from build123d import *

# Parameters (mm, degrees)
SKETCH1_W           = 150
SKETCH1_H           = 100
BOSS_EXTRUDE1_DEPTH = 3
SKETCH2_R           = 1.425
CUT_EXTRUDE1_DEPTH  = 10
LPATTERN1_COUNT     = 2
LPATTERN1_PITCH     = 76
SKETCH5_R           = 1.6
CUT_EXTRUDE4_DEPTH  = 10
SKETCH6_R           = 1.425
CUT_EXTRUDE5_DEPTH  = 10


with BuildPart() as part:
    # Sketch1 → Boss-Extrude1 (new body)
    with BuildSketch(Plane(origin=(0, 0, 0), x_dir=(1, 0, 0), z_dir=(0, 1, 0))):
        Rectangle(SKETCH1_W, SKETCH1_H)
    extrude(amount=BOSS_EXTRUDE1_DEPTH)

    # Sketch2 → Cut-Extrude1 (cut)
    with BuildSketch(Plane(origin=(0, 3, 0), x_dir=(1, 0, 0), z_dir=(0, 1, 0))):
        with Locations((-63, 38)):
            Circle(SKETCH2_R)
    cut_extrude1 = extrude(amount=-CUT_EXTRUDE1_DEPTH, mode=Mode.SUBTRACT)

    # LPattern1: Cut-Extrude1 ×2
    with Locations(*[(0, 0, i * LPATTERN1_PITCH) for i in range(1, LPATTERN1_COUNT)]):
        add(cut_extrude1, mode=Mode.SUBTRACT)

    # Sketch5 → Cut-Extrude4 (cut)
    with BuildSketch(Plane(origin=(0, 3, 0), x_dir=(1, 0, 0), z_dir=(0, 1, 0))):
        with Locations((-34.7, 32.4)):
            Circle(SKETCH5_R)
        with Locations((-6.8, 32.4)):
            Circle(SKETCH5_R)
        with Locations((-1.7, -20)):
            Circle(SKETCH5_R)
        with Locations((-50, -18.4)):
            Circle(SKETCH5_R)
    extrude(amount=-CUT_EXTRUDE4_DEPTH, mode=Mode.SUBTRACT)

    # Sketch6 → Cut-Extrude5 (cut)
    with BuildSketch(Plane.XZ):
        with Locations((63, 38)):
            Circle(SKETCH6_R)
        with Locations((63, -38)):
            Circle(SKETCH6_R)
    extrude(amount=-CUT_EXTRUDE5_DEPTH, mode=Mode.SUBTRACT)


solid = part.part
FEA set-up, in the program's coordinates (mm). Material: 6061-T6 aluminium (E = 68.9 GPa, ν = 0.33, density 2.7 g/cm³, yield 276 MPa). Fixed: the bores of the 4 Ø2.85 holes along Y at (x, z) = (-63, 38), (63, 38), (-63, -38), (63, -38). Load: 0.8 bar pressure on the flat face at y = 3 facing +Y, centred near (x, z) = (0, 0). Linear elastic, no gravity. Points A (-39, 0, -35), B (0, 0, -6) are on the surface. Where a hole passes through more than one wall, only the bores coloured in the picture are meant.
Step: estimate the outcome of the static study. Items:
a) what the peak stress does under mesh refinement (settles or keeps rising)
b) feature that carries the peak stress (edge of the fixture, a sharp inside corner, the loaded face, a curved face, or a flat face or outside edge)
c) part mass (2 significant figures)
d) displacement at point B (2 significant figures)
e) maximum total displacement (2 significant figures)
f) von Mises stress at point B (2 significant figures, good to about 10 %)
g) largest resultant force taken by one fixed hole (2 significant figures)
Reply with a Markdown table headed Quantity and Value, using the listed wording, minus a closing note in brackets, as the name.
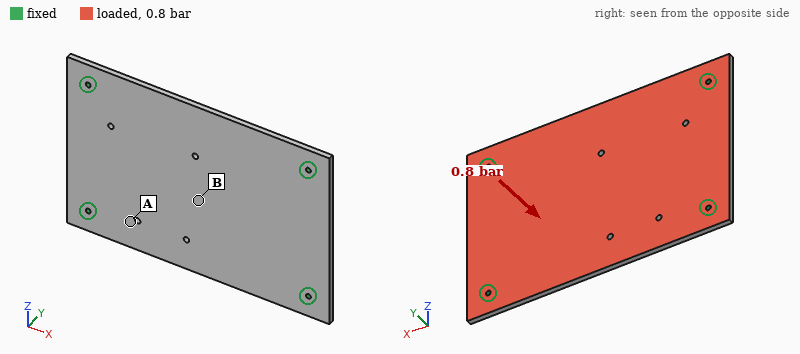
| Quantity | Value |
|---|---|
| what the peak stress does under mesh refinement | keeps rising |
| feature that carries the peak stress | edge of the fixture |
| part mass | 120 g |
| displacement at point B | 0.51 mm |
| maximum total displacement | 0.51 mm |
| von Mises stress at point B | 37 MPa |
| largest resultant force taken by one fixed hole | 300 N |
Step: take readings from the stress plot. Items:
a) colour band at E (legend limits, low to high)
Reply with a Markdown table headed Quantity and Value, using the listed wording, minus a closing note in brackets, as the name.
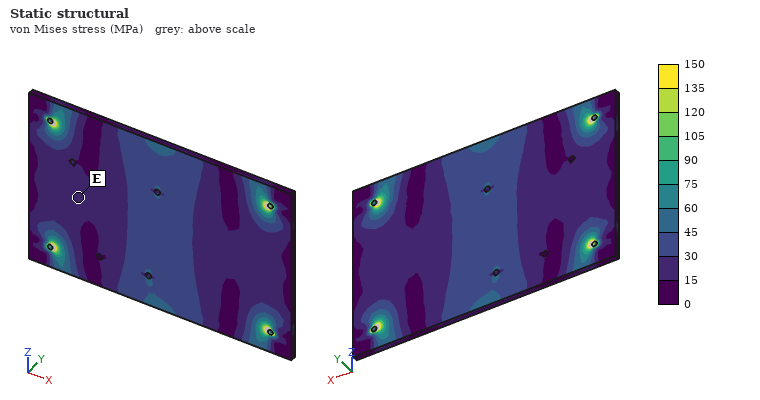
| Quantity | Value |
|---|---|
| colour band at E | 15 to 30 MPa |
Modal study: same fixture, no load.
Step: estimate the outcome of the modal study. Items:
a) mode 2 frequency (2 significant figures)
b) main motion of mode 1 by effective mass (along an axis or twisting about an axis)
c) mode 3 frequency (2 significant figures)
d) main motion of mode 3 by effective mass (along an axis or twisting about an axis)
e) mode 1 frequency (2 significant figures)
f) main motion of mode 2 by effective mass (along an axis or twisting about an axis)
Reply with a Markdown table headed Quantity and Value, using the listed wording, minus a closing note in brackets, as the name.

| Quantity | Value |
|---|---|
| mode 2 frequency | 1200 Hz |
| main motion of mode 1 by effective mass | along Y |
| mode 3 frequency | 2100 Hz |
| main motion of mode 3 by effective mass | twisting about Z |
| mode 1 frequency | 810 Hz |
| main motion of mode 2 by effective mass | twisting about X |
